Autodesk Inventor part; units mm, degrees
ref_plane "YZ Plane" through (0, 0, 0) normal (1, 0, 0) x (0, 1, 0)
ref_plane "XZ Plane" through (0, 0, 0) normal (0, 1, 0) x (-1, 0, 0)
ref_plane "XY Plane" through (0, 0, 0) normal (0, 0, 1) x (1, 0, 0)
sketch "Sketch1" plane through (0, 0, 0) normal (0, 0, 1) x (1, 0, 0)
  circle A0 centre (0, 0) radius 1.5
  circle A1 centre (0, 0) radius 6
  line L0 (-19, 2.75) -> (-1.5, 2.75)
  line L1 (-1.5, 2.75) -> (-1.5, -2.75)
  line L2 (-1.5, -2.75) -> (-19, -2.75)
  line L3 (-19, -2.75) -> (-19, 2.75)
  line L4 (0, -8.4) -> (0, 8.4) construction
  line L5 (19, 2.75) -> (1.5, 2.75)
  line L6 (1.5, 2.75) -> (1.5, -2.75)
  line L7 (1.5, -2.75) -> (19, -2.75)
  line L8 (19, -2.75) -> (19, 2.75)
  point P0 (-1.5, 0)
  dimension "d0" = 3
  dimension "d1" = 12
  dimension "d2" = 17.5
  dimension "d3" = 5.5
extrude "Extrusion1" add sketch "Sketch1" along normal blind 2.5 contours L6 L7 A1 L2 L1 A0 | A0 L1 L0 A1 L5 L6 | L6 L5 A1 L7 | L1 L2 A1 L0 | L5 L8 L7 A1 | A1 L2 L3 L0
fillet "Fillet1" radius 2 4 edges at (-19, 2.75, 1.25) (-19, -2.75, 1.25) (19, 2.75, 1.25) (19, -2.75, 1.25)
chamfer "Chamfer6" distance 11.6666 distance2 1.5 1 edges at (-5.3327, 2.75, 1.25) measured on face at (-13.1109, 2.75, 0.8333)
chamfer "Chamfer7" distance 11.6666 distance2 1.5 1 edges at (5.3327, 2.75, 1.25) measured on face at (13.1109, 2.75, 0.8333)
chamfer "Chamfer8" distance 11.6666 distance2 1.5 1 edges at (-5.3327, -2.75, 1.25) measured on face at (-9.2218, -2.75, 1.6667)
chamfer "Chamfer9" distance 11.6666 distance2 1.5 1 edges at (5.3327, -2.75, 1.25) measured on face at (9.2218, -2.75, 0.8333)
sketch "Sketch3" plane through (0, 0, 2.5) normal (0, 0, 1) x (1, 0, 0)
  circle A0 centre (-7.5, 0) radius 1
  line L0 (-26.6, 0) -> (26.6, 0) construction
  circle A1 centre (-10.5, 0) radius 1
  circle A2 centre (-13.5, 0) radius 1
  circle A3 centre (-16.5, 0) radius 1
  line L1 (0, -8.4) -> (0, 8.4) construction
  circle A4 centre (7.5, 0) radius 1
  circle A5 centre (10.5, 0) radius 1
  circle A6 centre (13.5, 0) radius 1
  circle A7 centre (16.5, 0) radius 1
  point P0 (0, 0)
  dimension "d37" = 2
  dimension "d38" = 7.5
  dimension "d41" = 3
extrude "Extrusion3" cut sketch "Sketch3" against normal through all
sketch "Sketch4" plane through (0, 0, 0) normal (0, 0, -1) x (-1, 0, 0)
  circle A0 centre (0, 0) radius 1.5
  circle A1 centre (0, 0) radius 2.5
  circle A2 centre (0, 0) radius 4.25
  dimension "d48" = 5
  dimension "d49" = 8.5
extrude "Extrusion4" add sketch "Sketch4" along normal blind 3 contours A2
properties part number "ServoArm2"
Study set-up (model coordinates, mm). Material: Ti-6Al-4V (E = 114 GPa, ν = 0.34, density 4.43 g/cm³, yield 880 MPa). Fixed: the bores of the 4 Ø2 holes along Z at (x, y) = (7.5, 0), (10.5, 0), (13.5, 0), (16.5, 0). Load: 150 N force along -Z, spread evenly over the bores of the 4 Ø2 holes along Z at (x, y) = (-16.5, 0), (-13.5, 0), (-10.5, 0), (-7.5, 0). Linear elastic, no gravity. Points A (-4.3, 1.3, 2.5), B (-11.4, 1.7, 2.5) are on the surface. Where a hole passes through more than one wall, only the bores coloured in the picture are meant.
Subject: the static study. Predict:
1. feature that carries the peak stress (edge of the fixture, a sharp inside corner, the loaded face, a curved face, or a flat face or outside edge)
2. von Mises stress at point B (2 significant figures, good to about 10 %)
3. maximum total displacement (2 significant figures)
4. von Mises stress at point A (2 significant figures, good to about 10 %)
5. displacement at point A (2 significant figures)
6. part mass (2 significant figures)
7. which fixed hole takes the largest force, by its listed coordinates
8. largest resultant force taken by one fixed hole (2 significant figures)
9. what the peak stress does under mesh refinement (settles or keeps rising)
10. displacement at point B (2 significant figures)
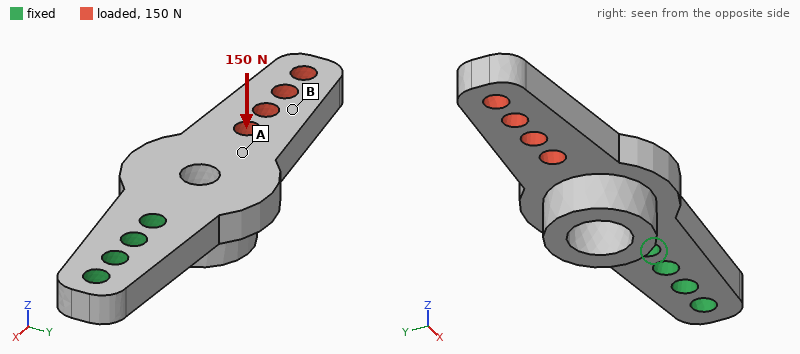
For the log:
edge of the fixture
56 MPa
0.37 mm
120 MPa
0.11 mm
3.3 g
(7.5, 0)
360 N
keeps rising
0.23 mm
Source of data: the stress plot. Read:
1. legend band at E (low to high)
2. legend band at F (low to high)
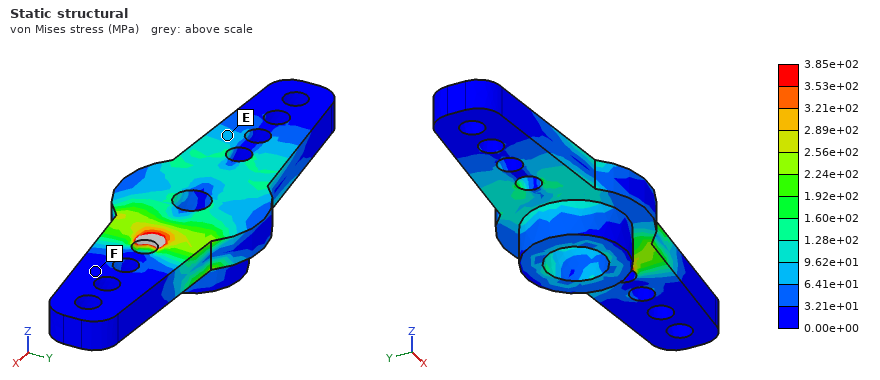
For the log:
6.41e+01 to 9.62e+01 MPa
0.00e+00 to 3.21e+01 MPa
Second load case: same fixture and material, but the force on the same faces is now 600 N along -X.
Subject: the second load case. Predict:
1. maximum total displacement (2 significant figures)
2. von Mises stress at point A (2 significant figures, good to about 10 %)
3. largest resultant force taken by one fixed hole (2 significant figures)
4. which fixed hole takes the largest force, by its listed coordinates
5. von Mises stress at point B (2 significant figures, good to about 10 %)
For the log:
12 µm
25 MPa
450 N
(7.5, 0)
27 MPa
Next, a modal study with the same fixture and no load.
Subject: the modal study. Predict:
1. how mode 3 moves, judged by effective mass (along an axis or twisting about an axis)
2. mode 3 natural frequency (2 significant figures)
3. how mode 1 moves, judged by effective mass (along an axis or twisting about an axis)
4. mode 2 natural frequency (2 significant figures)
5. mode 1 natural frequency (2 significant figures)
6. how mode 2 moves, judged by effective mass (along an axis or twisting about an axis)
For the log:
along Z
17 kHz
along Z
8900 Hz
4100 Hz
along Y
